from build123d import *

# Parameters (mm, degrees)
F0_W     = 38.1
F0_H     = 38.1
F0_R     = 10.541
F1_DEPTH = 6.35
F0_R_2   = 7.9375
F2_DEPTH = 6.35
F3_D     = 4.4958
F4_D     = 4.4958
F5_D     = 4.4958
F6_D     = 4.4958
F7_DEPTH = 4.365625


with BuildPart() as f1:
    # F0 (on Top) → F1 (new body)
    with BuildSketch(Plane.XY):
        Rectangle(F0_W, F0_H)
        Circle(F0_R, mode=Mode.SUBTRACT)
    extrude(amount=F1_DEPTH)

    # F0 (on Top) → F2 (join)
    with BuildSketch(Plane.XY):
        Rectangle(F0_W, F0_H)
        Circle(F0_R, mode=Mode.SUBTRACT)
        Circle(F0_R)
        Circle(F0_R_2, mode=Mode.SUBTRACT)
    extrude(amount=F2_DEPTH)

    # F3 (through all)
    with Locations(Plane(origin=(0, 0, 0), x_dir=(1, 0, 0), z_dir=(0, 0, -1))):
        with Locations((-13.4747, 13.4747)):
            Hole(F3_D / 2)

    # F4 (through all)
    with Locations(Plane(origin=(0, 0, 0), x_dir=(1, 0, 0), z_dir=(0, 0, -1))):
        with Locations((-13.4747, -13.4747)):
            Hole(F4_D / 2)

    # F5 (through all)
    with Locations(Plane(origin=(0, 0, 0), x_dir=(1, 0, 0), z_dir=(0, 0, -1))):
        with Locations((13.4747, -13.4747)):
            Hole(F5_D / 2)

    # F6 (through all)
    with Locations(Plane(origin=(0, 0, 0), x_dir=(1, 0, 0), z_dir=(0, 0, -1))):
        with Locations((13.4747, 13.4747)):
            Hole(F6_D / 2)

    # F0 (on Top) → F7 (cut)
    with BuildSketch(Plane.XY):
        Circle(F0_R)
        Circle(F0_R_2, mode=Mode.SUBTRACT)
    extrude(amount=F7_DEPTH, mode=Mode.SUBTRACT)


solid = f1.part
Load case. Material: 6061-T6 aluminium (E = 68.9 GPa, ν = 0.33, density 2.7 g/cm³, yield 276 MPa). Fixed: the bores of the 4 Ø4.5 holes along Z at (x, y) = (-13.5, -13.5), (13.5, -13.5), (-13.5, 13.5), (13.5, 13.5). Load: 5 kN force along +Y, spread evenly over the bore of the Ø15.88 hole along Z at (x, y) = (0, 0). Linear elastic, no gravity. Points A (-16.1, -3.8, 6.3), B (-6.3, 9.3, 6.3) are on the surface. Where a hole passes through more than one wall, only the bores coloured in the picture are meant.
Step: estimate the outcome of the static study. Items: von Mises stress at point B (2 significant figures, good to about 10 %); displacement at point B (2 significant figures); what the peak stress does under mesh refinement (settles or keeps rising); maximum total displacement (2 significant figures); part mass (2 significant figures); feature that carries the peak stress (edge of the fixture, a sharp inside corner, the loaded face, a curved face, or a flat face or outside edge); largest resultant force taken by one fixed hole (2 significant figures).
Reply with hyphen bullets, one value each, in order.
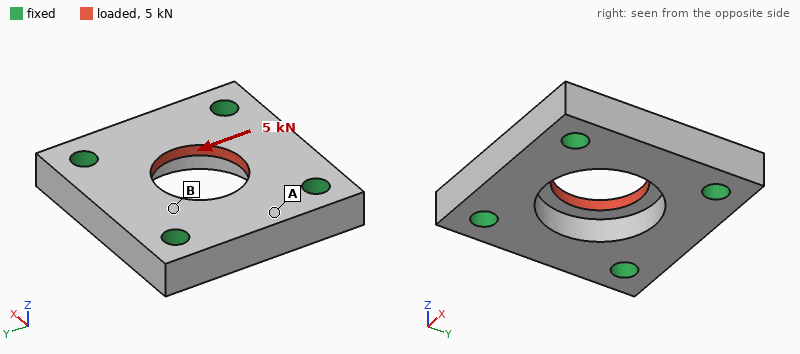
- 51 MPa
- 6.3 µm
- keeps rising
- 13 µm
- 19 g
- edge of the fixture
- 1.3 kN
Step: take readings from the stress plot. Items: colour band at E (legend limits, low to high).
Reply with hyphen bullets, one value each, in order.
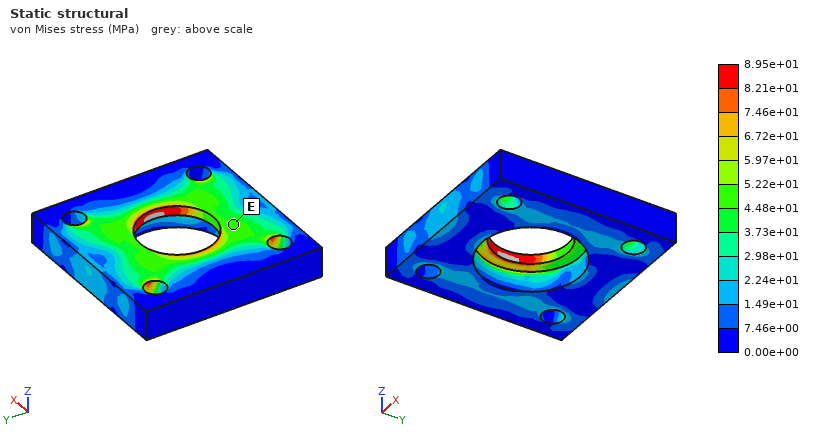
- 4.48e+01 to 5.22e+01 MPa
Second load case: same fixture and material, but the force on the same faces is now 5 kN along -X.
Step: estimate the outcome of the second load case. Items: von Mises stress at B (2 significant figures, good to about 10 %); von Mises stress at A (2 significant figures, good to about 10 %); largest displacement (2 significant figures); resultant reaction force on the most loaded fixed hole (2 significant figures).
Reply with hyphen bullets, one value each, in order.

- 41 MPa
- 22 MPa
- 13 µm
- 1.3 kN
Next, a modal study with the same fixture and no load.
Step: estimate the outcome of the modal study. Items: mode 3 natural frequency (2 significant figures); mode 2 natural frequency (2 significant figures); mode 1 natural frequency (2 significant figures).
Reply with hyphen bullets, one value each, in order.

- 41 kHz
- 39 kHz
- 39 kHz
